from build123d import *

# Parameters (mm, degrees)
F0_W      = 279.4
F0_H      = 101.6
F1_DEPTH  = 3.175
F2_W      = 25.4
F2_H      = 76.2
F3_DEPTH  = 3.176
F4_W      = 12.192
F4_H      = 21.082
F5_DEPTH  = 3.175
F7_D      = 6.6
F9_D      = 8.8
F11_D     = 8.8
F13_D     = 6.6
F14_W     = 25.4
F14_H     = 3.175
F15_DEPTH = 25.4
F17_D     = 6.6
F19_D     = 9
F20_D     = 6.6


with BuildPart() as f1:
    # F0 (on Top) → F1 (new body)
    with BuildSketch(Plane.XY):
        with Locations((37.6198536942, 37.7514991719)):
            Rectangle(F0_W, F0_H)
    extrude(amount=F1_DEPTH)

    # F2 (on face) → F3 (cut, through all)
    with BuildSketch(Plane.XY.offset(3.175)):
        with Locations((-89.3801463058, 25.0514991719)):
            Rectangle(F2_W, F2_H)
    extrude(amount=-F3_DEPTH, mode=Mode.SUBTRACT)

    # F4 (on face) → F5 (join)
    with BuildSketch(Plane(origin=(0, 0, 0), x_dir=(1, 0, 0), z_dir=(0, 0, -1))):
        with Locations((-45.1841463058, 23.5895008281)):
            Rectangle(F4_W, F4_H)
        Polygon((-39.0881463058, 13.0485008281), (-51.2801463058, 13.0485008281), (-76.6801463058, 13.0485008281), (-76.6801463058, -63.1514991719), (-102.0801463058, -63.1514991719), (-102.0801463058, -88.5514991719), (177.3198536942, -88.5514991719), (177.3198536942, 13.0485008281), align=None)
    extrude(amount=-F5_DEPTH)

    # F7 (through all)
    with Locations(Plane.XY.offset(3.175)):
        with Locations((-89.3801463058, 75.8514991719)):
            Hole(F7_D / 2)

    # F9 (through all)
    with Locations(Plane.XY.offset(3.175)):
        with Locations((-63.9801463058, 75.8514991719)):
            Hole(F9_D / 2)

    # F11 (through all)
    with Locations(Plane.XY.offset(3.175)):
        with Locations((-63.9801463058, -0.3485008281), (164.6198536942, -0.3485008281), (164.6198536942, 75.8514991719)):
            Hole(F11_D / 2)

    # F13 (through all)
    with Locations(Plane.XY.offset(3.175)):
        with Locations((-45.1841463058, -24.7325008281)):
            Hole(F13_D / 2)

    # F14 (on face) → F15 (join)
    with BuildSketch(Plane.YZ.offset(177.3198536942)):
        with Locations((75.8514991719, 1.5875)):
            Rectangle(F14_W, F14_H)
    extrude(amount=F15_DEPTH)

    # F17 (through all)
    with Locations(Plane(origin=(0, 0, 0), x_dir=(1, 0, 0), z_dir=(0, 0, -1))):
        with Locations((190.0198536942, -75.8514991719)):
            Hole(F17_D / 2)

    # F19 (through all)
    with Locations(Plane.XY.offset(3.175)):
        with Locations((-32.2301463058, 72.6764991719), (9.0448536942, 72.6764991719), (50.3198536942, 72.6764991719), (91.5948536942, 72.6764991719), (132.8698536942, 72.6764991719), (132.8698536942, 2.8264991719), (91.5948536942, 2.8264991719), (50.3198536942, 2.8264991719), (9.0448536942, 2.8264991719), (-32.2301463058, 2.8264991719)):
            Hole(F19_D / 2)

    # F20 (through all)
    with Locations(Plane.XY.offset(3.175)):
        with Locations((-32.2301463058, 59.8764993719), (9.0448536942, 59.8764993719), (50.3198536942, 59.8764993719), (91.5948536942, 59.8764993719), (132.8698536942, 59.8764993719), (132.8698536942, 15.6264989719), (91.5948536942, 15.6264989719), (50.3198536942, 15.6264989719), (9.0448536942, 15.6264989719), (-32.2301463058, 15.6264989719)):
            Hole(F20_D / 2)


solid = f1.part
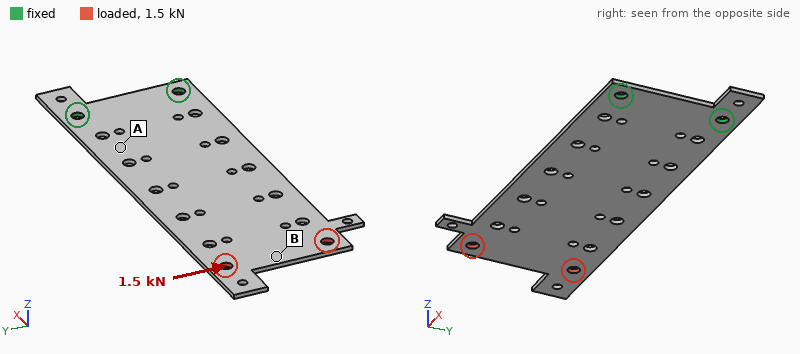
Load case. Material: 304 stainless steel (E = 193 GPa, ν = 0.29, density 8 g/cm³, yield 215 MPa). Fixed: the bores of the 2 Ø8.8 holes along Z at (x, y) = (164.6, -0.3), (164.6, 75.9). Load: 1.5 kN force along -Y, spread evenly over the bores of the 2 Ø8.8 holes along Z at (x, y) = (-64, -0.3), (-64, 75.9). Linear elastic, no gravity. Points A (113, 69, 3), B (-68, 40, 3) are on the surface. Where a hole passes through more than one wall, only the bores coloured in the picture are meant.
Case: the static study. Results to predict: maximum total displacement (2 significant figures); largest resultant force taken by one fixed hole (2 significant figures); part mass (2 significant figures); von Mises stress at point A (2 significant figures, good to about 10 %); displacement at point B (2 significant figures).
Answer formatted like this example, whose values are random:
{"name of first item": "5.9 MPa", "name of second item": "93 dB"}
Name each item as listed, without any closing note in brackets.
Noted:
{"maximum total displacement": "0.19 mm", "largest resultant force taken by one fixed hole": "4.4 kN", "part mass": "660 g", "von Mises stress at point A": "25 MPa", "displacement at point B": "0.15 mm"}
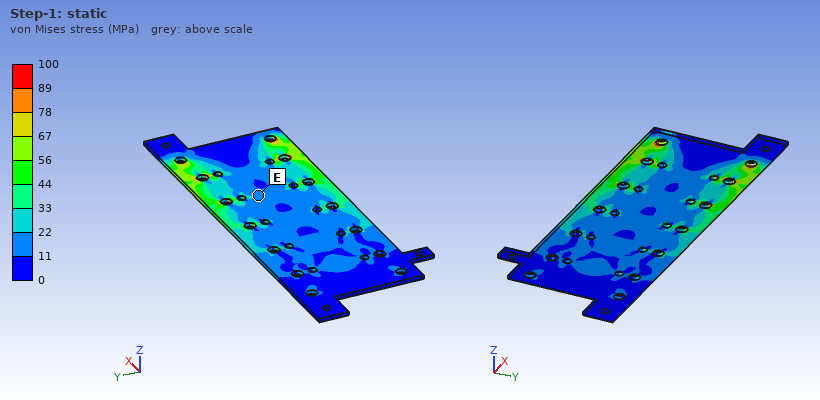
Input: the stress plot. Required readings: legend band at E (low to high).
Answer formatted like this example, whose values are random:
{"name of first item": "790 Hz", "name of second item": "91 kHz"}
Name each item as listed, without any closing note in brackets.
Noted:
{"legend band at E": "11 to 22 MPa"}
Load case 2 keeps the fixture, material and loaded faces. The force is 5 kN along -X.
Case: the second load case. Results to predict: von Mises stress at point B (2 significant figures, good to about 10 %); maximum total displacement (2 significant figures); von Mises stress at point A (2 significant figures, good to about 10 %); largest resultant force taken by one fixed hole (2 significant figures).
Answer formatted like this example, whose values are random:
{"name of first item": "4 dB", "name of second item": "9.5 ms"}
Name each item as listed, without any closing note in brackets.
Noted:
{"von Mises stress at point B": "11 MPa", "maximum total displacement": "27 µm", "von Mises stress at point A": "13 MPa", "largest resultant force taken by one fixed hole": "2.6 kN"}
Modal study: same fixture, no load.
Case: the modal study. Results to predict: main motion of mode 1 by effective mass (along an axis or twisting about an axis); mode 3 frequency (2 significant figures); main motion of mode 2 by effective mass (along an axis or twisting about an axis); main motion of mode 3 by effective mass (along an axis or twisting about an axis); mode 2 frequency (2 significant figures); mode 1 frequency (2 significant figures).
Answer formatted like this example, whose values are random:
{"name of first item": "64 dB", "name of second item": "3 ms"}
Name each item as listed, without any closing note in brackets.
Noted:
{"main motion of mode 1 by effective mass": "along Z", "mode 3 frequency": "250 Hz", "main motion of mode 2 by effective mass": "twisting about X", "main motion of mode 3 by effective mass": "along Z", "mode 2 frequency": "200 Hz", "mode 1 frequency": "39 Hz"}
